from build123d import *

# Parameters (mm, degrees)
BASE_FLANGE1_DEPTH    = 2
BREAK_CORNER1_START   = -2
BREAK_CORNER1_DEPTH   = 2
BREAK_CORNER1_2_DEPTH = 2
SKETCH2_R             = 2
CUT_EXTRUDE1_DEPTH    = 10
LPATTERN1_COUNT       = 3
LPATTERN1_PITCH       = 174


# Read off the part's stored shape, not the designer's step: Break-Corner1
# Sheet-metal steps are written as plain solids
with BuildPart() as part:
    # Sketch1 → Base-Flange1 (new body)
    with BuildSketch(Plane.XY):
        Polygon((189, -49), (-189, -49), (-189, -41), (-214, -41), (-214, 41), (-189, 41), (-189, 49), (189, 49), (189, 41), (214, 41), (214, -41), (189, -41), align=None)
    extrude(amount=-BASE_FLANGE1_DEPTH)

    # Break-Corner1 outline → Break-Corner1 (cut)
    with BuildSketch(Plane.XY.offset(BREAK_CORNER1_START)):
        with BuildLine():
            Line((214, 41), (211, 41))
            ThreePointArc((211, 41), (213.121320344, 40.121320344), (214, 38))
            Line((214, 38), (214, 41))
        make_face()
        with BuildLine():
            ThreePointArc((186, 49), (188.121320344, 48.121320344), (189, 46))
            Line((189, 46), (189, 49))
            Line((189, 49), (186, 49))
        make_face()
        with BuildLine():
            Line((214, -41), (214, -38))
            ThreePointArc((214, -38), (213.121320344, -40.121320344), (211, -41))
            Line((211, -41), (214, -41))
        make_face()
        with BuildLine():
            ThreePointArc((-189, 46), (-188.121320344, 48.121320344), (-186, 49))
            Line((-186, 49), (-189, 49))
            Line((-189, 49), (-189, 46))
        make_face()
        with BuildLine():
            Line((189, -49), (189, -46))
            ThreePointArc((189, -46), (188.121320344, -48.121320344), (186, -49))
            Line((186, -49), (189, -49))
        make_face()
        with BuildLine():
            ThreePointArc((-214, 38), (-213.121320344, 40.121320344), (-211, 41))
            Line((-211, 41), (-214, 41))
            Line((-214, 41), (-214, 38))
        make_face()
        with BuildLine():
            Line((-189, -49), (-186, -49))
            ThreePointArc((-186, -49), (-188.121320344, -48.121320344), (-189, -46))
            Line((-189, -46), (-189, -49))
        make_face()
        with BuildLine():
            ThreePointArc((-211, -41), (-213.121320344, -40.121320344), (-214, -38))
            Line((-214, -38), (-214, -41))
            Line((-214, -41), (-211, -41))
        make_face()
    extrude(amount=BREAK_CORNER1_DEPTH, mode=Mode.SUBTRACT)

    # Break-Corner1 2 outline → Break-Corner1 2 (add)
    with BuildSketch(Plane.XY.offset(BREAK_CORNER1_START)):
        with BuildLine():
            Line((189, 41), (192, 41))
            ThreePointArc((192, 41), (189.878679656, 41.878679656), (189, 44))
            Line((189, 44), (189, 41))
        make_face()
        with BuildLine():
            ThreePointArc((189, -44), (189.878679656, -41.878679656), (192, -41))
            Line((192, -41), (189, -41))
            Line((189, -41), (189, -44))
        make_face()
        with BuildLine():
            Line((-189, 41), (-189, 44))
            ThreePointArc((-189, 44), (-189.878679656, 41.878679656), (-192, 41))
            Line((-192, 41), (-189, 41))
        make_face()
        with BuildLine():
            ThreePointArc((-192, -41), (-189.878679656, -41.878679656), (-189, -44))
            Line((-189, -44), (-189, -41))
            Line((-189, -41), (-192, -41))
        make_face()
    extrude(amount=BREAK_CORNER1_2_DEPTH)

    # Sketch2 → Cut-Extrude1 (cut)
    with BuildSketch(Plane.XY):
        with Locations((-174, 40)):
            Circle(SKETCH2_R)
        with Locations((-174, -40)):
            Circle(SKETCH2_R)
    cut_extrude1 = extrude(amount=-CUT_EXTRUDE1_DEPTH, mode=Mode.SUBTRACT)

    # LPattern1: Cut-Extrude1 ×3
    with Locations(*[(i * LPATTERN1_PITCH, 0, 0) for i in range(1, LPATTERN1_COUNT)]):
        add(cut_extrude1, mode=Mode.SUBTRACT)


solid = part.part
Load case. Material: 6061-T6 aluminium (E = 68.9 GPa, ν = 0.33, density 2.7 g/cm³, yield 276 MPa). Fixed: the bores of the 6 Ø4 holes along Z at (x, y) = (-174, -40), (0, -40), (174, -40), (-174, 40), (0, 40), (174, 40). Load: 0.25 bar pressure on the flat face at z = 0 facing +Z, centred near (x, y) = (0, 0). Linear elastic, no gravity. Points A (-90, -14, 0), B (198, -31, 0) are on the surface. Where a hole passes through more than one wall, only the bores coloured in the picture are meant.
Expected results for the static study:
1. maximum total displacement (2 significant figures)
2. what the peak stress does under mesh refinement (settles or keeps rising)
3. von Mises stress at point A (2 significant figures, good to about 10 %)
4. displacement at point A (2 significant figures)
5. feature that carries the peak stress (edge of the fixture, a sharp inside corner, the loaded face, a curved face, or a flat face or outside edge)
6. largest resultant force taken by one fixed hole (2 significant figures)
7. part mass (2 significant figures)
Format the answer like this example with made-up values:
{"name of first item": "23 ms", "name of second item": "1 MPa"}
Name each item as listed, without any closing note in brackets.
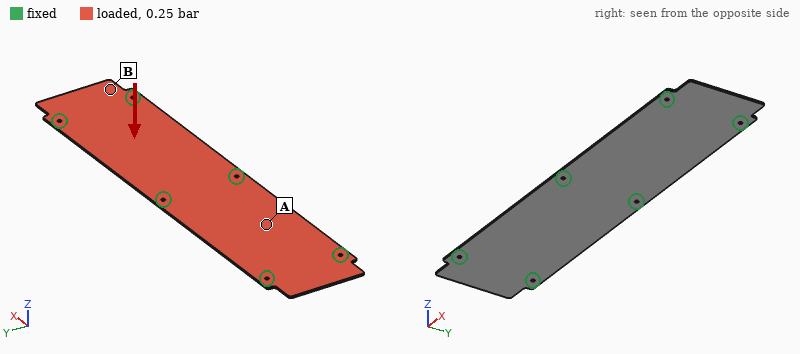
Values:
{"maximum total displacement": "1.4 mm", "what the peak stress does under mesh refinement": "keeps rising", "von Mises stress at point A": "43 MPa", "displacement at point A": "1.4 mm", "feature that carries the peak stress": "edge of the fixture", "largest resultant force taken by one fixed hole": "220 N", "part mass": "220 g"}
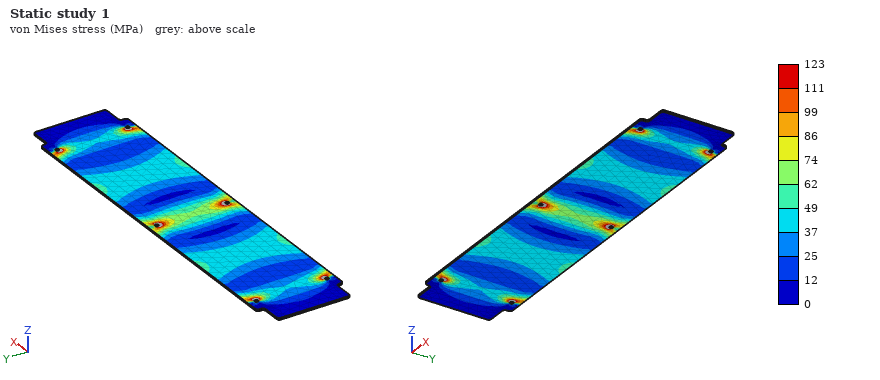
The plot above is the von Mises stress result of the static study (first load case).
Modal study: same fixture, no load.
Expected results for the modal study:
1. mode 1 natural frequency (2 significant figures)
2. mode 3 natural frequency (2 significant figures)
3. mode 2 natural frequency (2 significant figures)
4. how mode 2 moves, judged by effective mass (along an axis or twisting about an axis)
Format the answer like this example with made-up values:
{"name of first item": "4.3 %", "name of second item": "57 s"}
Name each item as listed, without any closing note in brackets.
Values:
{"mode 1 natural frequency": "300 Hz", "mode 3 natural frequency": "530 Hz", "mode 2 natural frequency": "330 Hz", "how mode 2 moves, judged by effective mass": "along Z"}
